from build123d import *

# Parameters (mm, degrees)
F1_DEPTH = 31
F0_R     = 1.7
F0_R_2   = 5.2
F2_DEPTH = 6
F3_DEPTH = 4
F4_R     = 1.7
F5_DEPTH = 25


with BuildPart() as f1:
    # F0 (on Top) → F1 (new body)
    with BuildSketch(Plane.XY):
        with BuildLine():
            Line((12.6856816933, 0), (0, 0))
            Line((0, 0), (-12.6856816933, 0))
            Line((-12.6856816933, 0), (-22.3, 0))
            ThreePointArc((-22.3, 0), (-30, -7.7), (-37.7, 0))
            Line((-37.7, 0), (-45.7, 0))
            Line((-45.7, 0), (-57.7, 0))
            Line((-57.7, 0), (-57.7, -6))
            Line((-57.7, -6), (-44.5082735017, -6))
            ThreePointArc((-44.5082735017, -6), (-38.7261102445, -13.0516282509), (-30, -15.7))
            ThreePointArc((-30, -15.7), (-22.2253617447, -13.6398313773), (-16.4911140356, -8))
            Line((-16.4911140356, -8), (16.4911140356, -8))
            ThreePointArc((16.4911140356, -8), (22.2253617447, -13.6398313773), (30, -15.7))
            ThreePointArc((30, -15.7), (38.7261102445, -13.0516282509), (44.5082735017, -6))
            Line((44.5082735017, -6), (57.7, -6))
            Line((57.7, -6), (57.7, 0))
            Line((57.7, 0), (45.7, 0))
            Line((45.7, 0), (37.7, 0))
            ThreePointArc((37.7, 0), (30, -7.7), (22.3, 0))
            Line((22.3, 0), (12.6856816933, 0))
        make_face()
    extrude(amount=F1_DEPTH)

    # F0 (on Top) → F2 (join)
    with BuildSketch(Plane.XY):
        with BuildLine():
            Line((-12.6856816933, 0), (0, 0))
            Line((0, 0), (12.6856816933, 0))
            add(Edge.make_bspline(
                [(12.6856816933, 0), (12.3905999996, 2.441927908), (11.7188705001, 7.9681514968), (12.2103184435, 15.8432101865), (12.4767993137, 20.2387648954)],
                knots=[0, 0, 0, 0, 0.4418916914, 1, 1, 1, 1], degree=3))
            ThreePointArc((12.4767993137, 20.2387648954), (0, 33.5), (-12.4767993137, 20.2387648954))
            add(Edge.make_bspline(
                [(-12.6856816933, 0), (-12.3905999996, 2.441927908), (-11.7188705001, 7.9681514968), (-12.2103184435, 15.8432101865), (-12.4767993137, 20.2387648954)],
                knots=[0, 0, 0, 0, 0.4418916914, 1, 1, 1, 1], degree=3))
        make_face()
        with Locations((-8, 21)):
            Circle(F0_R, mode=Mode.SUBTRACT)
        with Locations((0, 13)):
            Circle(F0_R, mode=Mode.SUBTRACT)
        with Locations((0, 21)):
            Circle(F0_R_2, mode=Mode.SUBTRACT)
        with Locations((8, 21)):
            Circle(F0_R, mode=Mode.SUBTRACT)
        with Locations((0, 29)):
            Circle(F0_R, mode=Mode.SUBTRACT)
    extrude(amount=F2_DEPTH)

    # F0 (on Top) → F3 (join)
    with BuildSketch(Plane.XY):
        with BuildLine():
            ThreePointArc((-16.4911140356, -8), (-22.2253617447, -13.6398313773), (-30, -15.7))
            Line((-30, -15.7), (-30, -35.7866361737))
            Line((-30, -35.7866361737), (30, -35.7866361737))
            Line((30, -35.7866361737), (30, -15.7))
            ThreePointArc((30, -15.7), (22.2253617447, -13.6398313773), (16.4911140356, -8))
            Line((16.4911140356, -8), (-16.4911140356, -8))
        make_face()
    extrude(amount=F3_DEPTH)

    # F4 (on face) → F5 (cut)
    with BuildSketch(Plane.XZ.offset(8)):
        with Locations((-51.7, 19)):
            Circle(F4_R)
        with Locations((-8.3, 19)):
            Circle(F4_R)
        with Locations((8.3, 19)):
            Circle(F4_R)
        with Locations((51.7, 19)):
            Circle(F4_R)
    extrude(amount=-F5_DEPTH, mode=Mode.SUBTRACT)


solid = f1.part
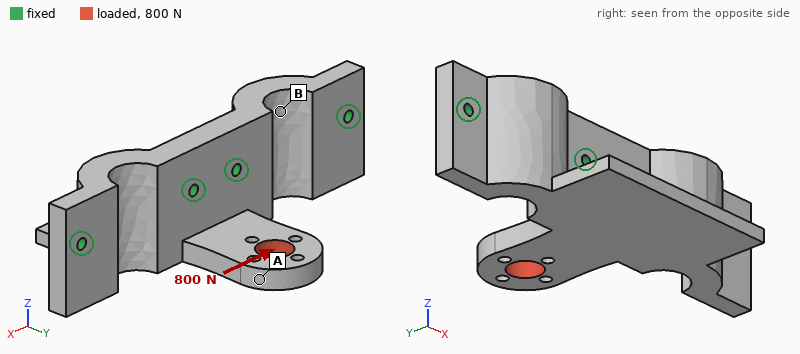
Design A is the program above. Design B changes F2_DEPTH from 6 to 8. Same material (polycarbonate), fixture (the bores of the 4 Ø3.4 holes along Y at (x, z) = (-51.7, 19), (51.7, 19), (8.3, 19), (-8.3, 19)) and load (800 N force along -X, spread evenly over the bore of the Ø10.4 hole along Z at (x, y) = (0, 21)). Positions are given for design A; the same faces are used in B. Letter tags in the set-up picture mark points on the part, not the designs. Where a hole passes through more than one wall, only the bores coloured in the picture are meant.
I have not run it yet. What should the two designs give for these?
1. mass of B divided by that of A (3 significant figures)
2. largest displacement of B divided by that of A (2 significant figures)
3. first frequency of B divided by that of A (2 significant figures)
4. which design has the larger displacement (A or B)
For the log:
1.03
0.80
1.0
A
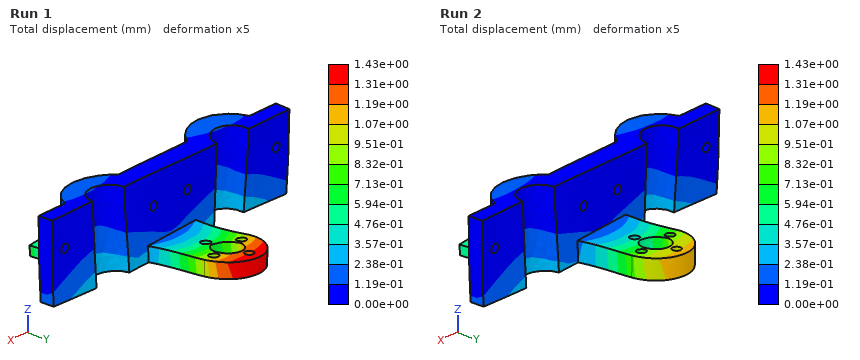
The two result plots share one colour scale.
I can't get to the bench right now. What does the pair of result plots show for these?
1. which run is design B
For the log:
Run 2
